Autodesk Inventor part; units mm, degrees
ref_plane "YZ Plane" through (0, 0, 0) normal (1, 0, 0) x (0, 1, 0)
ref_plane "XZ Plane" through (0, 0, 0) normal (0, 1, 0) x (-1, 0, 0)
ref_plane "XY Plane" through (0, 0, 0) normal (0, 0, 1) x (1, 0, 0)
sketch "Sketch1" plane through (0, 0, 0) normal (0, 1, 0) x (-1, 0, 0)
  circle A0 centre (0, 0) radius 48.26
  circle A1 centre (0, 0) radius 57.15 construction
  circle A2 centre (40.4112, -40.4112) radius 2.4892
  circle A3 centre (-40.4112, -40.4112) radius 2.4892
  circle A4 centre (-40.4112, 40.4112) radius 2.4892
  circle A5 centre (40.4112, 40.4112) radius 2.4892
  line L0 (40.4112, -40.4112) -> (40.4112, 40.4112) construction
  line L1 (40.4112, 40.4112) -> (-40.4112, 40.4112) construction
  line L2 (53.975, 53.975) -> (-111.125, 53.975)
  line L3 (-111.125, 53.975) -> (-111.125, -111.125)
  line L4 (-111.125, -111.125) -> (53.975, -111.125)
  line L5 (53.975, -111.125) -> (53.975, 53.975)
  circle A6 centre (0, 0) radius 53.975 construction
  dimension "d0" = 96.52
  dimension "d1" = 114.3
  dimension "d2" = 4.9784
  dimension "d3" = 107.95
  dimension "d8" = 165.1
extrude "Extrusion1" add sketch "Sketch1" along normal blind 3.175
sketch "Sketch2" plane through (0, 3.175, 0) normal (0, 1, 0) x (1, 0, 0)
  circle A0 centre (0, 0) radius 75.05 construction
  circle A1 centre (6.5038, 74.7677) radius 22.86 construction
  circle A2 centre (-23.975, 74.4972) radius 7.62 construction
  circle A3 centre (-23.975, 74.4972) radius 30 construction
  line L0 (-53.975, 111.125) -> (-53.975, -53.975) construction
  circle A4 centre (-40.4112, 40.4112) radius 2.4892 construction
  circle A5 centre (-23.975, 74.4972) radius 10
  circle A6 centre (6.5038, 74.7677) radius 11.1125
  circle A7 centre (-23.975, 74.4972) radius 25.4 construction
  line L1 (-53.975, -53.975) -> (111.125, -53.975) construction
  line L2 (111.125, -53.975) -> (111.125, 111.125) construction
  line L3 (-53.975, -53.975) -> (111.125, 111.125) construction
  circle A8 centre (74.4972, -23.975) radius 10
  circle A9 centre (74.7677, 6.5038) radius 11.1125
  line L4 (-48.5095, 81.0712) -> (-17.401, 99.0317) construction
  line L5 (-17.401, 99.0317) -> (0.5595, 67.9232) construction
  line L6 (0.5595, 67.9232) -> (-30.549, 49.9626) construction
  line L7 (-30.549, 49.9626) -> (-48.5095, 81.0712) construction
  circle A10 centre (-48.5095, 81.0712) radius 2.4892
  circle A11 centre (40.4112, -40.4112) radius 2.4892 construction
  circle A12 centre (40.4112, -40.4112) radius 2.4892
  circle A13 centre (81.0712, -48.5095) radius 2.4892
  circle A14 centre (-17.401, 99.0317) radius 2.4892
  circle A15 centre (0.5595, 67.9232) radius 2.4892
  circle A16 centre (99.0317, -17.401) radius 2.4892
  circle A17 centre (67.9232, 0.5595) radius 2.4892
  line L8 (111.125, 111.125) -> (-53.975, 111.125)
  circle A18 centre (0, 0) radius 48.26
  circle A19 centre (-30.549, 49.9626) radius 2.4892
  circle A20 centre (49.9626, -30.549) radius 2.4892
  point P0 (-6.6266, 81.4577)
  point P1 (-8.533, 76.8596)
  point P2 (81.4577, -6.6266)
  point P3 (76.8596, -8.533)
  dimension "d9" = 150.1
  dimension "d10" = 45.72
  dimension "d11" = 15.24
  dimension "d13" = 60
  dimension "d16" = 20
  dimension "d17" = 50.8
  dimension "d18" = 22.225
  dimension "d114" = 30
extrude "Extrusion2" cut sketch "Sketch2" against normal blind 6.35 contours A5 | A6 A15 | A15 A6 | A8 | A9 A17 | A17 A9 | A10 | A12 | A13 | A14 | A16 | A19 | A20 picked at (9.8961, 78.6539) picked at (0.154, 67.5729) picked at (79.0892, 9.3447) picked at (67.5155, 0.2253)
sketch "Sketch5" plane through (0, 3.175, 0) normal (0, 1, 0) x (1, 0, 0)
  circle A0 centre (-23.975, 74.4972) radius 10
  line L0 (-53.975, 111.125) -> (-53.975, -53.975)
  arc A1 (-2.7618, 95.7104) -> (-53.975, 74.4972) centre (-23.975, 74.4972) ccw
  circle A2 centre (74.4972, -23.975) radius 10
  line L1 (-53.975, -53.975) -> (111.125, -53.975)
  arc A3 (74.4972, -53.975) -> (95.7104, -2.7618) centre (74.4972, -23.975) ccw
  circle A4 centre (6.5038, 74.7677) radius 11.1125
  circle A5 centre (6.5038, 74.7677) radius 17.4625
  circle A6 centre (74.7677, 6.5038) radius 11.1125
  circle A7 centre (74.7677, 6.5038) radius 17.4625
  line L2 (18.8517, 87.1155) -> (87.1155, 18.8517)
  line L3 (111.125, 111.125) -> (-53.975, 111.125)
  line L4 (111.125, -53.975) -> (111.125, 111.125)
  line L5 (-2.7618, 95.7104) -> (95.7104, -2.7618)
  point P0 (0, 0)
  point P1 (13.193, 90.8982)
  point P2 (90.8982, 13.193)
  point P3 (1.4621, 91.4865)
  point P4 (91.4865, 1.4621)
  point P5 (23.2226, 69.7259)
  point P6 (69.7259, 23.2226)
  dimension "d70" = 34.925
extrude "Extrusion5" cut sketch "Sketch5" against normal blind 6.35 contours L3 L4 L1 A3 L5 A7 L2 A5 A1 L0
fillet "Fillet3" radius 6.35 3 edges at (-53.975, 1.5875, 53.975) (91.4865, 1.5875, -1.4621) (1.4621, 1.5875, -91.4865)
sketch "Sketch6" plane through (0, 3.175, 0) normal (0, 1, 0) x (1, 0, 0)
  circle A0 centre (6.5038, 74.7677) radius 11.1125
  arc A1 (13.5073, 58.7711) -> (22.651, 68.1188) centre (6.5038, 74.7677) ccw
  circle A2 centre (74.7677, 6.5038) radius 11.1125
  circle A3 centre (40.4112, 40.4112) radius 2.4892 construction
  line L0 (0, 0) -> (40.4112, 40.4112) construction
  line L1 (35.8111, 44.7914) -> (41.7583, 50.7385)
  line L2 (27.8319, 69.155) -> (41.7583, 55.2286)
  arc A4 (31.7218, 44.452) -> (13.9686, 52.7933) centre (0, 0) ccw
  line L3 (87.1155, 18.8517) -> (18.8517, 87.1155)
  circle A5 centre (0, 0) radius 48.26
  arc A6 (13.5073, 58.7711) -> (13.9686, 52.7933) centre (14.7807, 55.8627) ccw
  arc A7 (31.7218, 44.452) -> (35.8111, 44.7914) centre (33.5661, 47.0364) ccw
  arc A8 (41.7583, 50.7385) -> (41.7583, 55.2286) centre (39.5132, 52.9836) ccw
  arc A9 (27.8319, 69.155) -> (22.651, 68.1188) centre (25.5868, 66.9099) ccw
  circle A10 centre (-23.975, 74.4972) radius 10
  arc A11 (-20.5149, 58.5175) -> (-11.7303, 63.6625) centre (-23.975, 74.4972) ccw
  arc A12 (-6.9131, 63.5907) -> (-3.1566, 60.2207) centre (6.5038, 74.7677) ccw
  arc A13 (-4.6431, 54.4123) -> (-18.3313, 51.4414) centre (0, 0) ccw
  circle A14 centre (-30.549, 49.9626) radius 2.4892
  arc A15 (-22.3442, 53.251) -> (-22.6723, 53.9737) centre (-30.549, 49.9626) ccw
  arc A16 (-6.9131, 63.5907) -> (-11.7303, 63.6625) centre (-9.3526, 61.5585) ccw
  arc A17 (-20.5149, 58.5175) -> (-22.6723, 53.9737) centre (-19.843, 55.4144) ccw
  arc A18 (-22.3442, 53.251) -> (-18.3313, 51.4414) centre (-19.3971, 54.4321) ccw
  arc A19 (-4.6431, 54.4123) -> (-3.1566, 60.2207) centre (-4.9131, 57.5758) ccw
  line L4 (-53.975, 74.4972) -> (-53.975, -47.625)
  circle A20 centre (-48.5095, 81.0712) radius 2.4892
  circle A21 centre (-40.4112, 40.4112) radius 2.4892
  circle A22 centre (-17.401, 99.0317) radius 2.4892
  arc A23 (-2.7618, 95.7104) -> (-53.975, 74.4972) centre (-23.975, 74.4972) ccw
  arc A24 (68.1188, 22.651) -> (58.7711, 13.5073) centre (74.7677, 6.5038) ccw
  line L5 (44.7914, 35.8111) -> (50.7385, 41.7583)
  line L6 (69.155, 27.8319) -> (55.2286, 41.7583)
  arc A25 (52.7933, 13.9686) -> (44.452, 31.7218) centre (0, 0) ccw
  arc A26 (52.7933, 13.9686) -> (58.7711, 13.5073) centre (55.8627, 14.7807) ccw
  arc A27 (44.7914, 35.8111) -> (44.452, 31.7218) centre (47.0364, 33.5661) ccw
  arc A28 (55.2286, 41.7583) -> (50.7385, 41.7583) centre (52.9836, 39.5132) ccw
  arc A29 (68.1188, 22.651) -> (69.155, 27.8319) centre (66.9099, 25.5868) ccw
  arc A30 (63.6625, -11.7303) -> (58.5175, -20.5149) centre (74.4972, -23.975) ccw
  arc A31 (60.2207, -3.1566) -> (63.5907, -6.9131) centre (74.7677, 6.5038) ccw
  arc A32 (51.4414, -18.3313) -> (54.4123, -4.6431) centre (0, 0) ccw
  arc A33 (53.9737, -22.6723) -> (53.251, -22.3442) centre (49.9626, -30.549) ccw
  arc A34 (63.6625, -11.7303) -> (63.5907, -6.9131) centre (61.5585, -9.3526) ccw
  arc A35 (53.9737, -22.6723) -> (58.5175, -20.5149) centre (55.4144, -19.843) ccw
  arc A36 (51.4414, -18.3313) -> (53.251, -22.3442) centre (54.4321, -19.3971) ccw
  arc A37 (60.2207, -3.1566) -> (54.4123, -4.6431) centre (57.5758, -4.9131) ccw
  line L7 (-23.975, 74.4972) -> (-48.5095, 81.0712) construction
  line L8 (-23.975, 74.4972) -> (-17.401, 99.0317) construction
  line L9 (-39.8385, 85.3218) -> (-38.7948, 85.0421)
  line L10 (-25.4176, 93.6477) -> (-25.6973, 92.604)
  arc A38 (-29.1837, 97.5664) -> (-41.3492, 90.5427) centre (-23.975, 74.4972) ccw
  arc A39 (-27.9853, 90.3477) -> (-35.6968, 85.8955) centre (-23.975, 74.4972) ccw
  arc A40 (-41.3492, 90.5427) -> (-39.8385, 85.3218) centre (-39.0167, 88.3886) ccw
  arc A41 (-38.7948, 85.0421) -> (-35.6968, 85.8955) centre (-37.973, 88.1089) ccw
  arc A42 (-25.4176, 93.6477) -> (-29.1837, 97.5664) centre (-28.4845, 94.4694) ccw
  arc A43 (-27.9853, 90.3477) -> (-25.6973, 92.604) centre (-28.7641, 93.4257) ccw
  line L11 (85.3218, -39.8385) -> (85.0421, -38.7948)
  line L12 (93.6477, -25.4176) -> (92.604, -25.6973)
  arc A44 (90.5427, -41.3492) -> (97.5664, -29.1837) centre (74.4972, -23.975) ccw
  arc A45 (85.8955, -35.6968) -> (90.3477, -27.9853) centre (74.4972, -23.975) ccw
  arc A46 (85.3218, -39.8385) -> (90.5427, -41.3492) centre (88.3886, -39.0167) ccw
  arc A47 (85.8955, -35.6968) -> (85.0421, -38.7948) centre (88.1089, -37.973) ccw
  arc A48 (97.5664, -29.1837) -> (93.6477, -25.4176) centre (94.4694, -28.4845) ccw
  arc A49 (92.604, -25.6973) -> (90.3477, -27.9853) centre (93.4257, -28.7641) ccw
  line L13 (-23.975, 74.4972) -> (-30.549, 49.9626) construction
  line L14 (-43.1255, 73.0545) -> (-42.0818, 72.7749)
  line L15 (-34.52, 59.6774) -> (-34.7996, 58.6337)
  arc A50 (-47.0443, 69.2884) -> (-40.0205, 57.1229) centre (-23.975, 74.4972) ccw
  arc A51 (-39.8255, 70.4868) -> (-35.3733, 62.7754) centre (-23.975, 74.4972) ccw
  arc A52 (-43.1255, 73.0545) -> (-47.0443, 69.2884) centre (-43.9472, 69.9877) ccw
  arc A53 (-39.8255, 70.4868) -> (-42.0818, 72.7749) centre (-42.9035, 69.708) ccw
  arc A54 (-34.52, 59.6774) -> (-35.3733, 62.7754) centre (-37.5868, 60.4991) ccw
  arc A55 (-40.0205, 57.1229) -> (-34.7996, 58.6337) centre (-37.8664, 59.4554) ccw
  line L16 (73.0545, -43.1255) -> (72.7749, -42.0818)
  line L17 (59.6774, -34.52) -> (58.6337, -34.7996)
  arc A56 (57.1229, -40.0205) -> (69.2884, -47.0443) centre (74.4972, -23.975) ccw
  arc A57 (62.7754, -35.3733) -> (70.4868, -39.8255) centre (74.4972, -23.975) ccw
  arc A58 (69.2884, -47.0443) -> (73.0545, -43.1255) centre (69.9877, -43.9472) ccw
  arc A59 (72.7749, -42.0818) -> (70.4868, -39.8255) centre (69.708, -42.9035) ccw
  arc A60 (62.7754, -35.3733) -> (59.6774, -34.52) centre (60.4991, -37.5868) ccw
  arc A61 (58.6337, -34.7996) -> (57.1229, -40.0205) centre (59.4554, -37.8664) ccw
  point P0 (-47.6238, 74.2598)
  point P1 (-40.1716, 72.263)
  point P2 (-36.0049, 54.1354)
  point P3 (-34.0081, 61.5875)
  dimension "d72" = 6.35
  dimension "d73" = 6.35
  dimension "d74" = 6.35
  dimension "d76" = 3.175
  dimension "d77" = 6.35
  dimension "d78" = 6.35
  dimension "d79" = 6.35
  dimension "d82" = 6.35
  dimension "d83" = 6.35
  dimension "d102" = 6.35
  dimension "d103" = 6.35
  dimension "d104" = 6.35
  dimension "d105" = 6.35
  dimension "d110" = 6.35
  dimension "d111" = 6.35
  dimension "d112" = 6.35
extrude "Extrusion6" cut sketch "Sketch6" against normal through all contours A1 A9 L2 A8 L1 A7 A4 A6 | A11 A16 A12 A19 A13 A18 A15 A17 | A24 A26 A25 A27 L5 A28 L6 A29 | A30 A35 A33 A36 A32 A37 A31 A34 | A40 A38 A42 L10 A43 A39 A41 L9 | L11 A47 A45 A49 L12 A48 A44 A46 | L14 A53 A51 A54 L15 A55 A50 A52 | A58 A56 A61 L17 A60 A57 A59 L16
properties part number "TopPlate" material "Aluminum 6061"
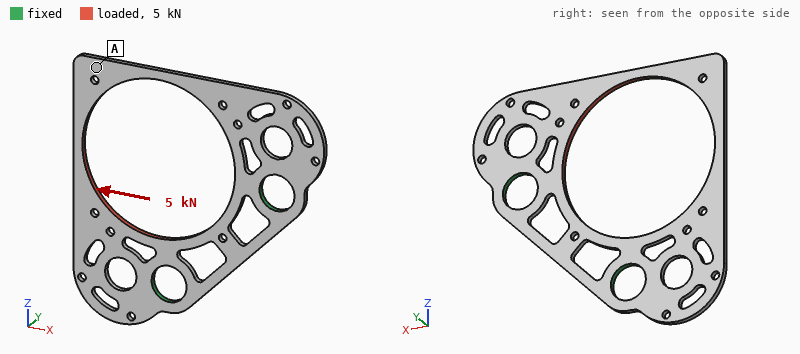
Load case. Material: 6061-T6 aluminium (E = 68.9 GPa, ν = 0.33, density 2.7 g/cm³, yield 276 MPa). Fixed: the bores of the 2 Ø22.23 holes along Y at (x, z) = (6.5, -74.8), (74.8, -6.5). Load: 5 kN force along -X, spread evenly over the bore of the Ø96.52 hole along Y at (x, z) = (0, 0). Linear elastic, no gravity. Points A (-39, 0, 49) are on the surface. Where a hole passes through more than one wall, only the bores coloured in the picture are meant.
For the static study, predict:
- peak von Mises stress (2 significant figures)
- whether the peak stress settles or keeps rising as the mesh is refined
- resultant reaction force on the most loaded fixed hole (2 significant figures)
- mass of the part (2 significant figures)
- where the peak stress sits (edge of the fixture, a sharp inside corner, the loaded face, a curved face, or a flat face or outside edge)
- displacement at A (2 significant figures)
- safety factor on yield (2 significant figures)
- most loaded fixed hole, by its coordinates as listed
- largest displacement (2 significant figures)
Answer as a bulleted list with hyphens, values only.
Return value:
- 300 MPa
- settles
- 2.8 kN
- 72 g
- a curved face
- 0.35 mm
- 0.92
- (74.8, -6.5)
- 0.50 mm
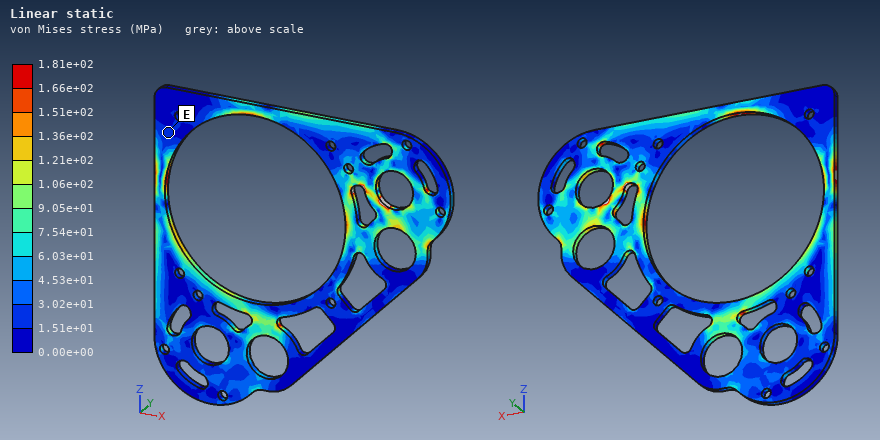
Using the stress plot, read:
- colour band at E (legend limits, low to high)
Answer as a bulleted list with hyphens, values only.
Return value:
- 1.51e+01 to 3.02e+01 MPa
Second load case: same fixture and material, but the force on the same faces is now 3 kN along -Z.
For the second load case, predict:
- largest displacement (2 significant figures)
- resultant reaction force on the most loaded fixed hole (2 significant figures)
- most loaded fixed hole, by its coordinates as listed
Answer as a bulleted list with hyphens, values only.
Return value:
- 0.30 mm
- 1.7 kN
- (6.5, -74.8)
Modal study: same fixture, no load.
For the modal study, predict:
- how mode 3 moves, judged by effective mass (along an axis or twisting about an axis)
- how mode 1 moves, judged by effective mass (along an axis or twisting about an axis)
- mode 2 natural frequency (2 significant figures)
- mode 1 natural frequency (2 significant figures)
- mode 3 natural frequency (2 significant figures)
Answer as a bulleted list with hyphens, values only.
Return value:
- along Y
- along Y
- 550 Hz
- 210 Hz
- 800 Hz
